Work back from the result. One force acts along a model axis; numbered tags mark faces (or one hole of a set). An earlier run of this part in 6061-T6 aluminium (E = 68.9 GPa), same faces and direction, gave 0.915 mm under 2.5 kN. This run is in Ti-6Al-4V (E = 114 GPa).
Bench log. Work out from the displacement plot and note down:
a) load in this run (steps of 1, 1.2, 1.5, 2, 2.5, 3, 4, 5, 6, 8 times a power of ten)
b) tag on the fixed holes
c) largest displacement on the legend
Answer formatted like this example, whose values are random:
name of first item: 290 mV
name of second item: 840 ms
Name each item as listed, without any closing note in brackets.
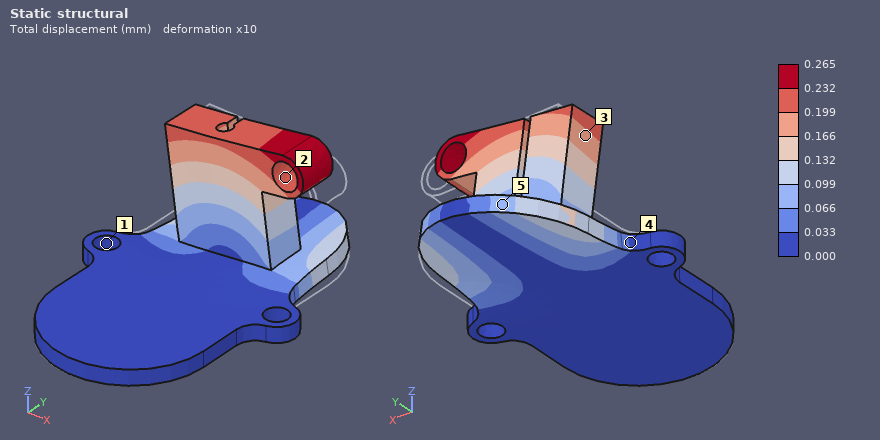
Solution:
load in this run: 1.2 kN
tag on the fixed holes: 1
largest displacement on the legend: 0.265 mm
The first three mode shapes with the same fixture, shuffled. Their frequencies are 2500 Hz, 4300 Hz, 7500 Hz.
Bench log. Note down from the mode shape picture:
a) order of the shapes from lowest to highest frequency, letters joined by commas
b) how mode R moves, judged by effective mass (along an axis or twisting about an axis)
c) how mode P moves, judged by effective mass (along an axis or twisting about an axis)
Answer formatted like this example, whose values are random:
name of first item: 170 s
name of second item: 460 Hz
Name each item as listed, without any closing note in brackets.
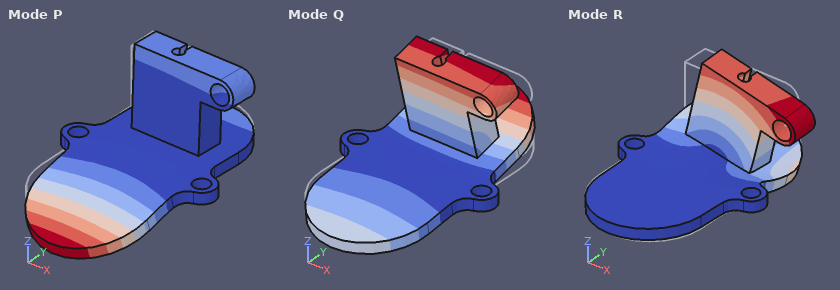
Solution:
order of the shapes from lowest to highest frequency, letters joined by commas: Q, P, R
how mode R moves, judged by effective mass: along X
how mode P moves, judged by effective mass: along Z
